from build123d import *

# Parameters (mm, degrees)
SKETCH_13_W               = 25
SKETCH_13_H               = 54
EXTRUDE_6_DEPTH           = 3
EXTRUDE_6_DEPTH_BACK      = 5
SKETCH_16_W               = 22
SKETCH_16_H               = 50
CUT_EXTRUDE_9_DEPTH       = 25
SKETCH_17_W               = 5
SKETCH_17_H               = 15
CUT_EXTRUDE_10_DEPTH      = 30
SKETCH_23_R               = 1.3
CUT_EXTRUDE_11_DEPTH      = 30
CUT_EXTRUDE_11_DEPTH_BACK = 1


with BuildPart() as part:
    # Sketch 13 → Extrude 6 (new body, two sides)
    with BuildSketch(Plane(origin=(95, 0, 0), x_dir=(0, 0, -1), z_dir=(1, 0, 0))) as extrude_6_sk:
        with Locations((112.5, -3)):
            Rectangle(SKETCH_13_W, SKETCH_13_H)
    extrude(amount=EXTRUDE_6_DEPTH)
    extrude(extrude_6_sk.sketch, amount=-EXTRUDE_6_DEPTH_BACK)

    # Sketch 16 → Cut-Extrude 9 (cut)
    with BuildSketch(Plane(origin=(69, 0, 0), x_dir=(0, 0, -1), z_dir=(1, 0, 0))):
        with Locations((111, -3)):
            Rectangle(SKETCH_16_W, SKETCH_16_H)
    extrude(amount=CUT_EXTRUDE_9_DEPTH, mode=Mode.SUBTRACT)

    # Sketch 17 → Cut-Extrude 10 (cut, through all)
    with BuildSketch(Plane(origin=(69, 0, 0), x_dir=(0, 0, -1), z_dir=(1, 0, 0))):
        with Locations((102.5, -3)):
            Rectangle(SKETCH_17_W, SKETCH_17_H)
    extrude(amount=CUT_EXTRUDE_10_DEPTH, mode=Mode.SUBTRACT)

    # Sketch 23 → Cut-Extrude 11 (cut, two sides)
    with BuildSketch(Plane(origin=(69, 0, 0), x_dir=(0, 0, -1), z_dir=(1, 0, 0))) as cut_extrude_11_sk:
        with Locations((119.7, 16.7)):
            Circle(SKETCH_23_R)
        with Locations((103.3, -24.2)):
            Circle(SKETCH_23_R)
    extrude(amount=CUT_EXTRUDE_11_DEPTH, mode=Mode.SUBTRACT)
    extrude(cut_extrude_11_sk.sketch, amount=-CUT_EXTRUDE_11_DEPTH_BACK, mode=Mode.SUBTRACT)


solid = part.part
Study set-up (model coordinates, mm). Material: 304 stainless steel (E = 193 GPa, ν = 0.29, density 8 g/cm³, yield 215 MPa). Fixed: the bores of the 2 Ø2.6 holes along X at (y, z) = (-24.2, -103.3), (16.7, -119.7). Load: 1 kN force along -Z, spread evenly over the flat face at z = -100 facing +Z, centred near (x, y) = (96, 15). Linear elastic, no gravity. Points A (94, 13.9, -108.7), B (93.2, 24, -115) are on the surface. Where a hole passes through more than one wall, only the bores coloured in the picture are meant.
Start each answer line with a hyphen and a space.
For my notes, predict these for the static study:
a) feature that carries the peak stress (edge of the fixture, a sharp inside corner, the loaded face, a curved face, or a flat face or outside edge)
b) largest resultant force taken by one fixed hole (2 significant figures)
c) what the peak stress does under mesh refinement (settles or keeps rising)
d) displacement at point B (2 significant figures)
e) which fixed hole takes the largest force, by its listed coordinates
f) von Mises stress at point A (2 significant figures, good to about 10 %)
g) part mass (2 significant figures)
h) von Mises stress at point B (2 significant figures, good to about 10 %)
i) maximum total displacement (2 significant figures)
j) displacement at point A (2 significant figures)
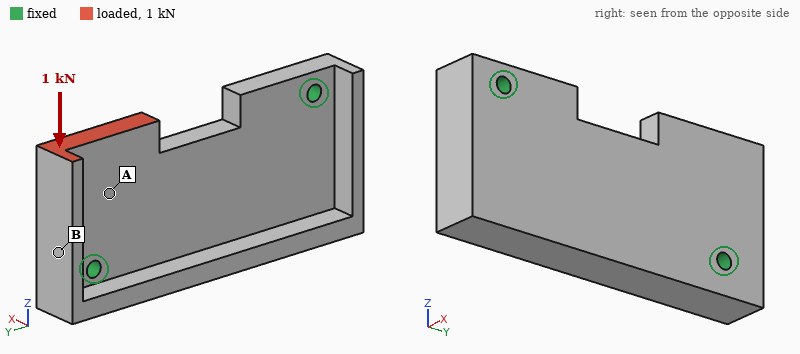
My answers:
- edge of the fixture
- 930 N
- keeps rising
- 1.2 µm
- (16.7, -119.7)
- 14 MPa
- 48 g
- 6.8 MPa
- 3.0 µm
- 1.4 µm
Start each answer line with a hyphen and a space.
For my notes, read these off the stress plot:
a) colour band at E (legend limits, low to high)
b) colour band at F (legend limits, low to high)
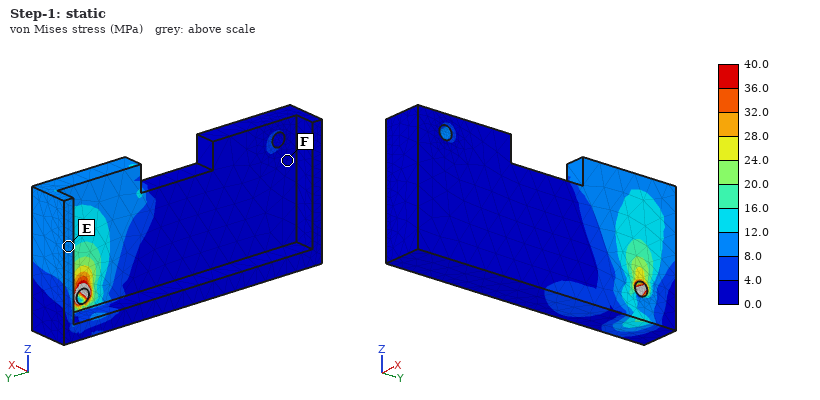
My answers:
- 8.0 to 12.0 MPa
- 0.0 to 4.0 MPa
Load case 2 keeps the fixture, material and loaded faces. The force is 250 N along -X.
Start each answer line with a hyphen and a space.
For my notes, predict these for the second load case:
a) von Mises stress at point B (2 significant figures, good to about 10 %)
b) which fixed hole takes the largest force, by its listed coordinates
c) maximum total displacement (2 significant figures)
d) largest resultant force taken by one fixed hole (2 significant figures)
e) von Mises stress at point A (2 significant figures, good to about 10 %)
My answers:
- 19 MPa
- (16.7, -119.7)
- 26 µm
- 220 N
- 21 MPa
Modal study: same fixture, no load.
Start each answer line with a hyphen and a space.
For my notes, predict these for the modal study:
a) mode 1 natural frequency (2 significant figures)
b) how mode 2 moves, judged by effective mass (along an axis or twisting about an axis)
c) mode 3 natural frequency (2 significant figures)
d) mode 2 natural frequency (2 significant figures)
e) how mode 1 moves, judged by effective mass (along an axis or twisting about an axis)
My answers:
- 5900 Hz
- along X
- 11 kHz
- 7800 Hz
- along X
